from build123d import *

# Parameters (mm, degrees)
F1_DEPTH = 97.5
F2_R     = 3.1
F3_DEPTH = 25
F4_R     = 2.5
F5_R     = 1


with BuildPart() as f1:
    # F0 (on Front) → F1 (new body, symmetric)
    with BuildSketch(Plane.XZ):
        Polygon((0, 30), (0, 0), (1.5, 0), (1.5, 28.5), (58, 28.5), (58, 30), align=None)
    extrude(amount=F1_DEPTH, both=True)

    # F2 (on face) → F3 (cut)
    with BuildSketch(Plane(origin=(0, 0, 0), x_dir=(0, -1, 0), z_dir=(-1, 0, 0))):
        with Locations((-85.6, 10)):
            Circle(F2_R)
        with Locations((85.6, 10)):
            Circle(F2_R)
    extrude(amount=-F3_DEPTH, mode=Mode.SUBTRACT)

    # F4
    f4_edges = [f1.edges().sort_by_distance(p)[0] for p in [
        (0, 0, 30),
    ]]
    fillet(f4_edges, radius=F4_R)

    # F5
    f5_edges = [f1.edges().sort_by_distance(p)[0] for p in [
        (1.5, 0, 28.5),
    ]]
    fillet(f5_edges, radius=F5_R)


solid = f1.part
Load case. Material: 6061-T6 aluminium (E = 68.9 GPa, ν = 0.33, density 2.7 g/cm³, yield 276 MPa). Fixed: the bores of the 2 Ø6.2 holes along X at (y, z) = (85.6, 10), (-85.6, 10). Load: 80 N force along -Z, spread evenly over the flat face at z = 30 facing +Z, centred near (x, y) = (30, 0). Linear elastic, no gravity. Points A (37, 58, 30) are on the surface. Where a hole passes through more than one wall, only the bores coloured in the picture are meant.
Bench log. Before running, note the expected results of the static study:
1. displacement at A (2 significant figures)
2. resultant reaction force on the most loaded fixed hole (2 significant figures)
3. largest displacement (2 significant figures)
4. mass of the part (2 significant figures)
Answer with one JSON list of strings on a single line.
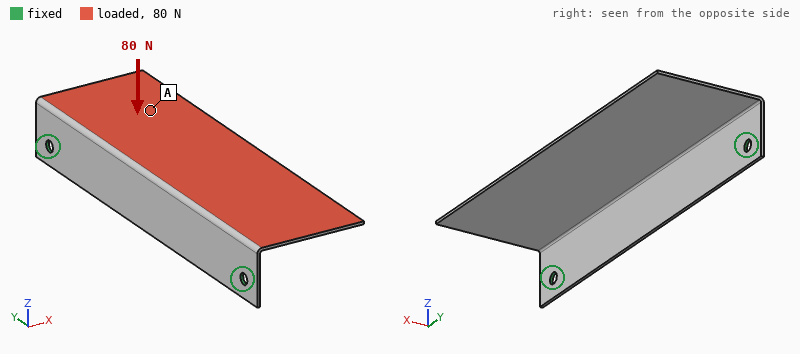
["1.3 mm", "51 N", "2.2 mm", "67 g"]
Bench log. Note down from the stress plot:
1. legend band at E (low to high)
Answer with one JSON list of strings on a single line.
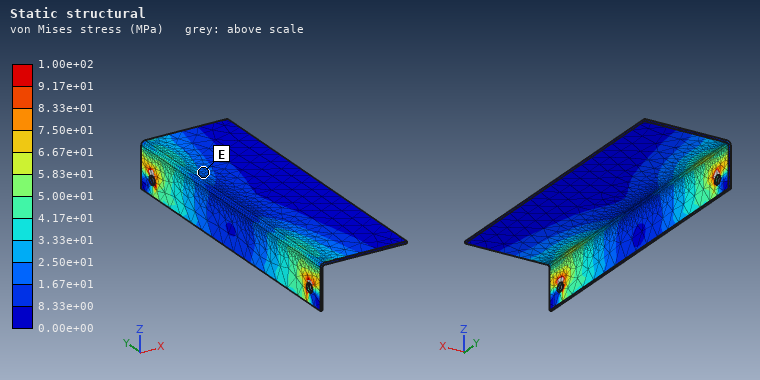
["1.67e+01 to 2.50e+01 MPa"]
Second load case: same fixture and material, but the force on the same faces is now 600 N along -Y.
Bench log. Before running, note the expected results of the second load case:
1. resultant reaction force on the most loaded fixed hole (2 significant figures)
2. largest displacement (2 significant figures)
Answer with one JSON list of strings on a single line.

["320 N", "0.72 mm"]
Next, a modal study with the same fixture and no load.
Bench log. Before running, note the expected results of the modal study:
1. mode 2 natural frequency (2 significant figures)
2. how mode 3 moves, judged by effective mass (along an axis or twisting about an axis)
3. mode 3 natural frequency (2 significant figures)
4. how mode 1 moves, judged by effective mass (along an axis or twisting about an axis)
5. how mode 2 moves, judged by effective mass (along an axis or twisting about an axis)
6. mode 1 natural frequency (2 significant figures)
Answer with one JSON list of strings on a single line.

["330 Hz", "along X", "510 Hz", "along Z", "twisting about X", "180 Hz"]
